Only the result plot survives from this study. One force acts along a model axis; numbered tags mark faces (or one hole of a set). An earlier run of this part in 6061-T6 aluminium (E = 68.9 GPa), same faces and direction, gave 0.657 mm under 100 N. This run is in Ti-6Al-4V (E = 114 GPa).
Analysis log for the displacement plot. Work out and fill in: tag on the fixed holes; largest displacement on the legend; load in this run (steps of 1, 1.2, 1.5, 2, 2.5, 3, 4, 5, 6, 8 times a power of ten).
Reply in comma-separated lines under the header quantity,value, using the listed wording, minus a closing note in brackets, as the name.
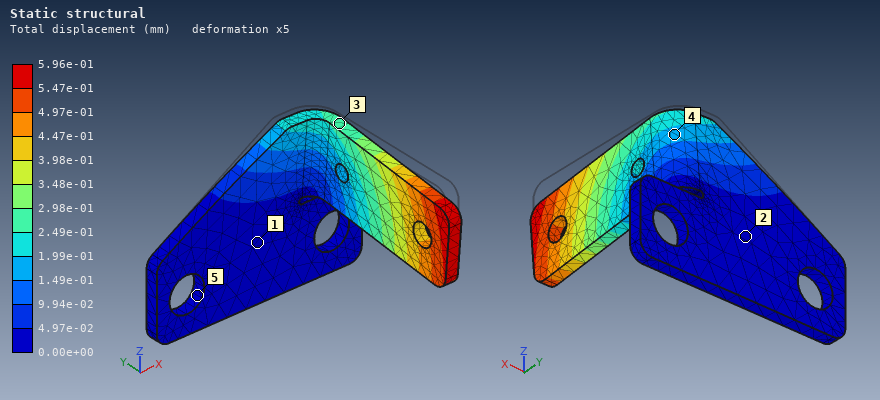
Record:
quantity,value
tag on the fixed holes,5
largest displacement on the legend,5.96e-01 mm
load in this run,150 N
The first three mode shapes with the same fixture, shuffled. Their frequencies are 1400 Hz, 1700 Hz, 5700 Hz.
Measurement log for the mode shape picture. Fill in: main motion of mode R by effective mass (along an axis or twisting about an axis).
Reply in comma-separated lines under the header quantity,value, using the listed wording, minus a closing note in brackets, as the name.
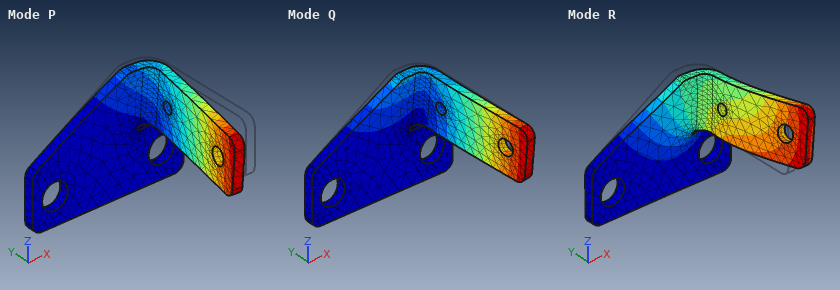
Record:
quantity,value
main motion of mode R by effective mass,along Y
